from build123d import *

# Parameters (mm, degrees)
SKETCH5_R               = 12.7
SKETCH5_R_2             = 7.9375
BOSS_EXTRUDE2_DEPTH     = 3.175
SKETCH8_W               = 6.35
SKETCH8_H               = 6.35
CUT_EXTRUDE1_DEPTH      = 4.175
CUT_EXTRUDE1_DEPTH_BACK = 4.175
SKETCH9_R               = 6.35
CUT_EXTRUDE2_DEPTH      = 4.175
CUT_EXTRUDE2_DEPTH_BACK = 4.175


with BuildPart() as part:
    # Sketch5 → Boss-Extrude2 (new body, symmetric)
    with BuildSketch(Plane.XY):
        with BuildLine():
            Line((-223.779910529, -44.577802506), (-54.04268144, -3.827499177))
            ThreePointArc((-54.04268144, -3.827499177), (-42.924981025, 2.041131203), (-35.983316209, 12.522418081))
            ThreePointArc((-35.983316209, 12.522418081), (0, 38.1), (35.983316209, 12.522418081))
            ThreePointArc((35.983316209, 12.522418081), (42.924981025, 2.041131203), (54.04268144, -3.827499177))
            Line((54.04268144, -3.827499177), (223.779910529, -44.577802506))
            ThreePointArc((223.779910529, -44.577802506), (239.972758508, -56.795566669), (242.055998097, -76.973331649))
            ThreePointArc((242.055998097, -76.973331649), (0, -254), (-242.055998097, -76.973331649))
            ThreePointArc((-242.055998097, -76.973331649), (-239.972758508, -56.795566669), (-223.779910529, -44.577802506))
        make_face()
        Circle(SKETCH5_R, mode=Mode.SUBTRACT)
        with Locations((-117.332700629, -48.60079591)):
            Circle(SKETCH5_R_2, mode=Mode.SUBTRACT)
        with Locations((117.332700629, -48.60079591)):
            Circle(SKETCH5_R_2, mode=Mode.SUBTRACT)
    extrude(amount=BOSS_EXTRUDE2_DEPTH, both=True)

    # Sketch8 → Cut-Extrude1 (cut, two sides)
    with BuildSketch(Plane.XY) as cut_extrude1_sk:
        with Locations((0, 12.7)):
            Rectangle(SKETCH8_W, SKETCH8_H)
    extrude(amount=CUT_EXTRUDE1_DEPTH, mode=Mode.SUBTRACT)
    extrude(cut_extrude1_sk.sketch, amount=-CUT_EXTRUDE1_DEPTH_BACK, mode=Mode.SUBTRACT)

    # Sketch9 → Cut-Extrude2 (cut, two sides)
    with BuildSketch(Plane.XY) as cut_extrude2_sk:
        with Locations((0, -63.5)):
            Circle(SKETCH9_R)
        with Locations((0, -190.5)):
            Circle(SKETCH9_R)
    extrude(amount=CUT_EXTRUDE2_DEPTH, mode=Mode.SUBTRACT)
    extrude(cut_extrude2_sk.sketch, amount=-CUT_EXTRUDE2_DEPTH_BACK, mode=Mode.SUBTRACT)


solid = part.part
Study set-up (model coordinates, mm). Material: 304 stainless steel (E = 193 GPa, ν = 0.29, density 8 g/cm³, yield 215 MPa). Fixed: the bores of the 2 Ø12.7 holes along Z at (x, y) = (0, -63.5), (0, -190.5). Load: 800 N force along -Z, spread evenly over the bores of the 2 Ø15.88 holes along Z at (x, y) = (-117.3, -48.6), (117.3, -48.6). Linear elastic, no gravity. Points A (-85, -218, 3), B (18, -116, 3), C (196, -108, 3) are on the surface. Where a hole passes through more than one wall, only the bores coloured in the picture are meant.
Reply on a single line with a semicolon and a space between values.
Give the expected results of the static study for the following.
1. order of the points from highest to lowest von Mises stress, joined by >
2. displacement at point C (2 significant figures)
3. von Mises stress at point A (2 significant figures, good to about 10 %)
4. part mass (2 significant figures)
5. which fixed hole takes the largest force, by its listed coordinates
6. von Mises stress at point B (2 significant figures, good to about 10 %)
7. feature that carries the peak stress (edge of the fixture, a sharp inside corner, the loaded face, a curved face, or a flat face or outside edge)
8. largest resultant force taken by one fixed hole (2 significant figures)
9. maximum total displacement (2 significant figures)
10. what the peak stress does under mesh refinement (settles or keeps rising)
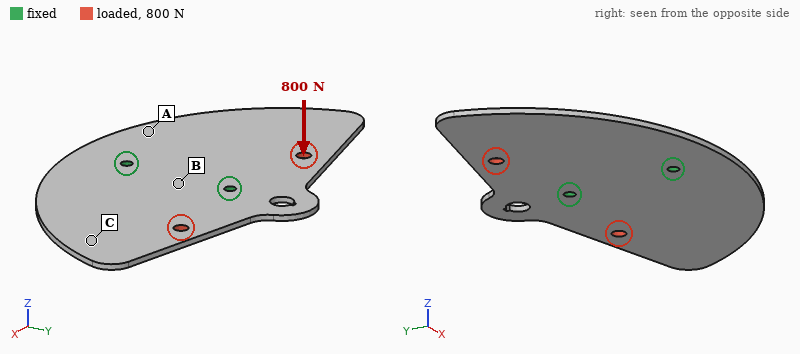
B > A > C; 0.41 mm; 9.9 MPa; 4.6 kg; (0, -63.5); 22 MPa; edge of the fixture; 810 N; 0.60 mm; keeps rising
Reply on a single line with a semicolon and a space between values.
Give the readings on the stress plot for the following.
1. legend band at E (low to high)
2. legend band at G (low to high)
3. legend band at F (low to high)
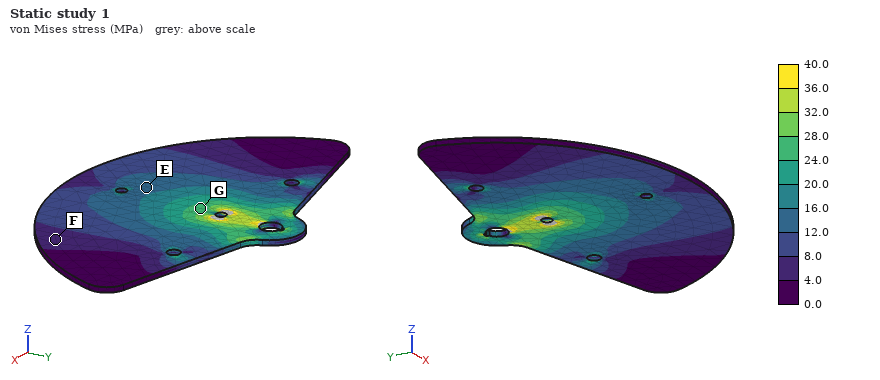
12.0 to 16.0 MPa; 24.0 to 28.0 MPa; 4.0 to 8.0 MPa
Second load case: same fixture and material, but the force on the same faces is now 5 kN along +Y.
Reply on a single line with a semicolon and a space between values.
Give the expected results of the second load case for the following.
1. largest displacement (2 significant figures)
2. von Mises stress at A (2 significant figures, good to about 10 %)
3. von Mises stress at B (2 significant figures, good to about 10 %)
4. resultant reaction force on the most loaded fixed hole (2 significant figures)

6.1 µm; 1.8 MPa; 2.3 MPa; 2.6 kN
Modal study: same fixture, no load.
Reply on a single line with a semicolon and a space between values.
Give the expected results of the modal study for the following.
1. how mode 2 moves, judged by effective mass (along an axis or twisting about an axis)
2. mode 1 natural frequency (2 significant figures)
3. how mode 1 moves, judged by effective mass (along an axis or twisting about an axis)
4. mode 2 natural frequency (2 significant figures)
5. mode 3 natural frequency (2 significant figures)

along Z; 110 Hz; twisting about Y; 130 Hz; 350 Hz
